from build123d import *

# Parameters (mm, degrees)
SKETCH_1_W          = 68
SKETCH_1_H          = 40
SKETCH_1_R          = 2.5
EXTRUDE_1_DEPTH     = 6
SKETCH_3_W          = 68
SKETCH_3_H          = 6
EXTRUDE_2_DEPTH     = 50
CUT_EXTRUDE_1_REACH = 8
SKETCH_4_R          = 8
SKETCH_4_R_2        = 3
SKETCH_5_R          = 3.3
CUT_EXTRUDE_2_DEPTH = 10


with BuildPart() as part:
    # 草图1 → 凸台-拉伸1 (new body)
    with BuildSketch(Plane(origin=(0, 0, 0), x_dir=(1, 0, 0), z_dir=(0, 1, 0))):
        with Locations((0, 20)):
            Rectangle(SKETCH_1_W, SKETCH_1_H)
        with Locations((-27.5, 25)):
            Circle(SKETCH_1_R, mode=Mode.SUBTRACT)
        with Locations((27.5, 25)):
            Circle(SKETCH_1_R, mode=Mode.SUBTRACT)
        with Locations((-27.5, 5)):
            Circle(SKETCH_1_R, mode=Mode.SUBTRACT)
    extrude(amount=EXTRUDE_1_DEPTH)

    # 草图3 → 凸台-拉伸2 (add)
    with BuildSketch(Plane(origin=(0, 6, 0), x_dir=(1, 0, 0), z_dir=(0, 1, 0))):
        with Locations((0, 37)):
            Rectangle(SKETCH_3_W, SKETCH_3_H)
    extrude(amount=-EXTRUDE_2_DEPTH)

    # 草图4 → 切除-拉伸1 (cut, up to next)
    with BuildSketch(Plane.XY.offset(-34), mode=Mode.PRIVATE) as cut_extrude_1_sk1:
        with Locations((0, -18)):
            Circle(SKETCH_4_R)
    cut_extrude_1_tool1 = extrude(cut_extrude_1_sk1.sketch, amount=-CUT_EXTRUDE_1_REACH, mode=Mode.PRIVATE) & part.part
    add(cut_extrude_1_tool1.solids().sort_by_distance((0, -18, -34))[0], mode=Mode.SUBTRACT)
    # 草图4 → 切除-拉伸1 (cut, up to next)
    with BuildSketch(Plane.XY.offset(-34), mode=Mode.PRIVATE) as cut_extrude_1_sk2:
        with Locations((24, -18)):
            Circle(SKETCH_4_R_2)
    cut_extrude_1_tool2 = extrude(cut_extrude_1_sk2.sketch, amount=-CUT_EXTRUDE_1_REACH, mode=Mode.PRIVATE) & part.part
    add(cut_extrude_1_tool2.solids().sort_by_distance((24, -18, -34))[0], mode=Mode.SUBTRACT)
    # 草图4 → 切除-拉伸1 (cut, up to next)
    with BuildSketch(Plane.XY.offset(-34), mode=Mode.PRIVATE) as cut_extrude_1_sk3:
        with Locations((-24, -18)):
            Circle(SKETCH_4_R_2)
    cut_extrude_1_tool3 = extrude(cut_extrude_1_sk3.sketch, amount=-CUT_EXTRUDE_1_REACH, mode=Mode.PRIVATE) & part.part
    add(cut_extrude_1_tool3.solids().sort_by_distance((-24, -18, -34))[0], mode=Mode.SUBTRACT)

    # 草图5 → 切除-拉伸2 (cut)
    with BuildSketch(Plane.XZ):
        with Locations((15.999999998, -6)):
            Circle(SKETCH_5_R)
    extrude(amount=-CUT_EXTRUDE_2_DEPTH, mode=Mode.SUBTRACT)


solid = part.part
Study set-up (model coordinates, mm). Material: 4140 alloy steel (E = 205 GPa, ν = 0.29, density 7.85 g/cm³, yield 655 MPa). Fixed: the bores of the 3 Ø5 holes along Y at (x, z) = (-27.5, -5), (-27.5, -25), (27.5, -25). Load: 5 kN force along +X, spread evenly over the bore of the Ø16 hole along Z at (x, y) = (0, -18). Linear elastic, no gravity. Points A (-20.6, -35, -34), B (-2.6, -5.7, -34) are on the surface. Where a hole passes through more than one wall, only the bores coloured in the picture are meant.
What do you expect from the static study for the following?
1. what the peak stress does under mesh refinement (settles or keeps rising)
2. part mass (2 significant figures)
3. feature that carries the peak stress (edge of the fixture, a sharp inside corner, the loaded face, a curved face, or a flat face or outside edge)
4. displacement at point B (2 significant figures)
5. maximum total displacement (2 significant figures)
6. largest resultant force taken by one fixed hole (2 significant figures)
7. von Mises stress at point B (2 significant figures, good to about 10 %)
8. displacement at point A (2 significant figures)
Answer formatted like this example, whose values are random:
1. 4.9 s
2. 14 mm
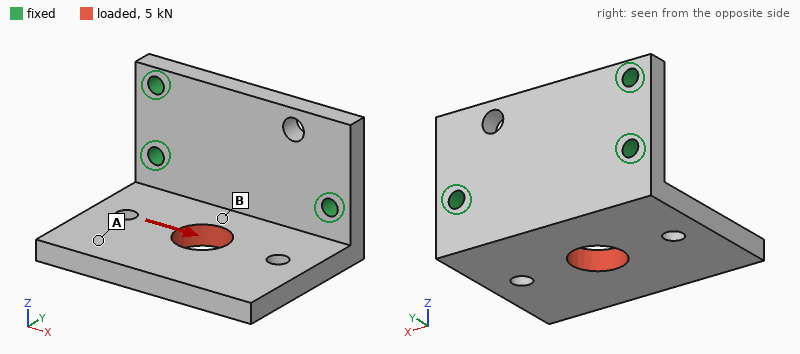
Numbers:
1. keeps rising
2. 250 g
3. edge of the fixture
4. 7.9 µm
5. 39 µm
6. 3.2 kN
7. 59 MPa
8. 29 µm
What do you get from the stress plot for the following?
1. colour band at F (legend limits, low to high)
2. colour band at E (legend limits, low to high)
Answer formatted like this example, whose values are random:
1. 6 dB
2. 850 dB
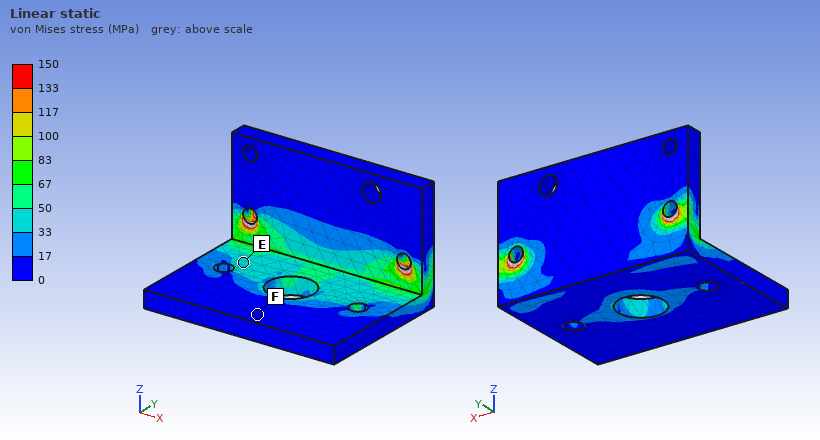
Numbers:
1. 0 to 17 MPa
2. 33 to 50 MPa
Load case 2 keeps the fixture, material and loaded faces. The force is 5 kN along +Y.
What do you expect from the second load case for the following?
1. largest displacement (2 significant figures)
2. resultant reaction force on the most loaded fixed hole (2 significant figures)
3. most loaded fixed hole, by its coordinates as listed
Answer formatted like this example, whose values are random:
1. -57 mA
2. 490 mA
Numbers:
1. 95 µm
2. 3.0 kN
3. (-27.5, -25)
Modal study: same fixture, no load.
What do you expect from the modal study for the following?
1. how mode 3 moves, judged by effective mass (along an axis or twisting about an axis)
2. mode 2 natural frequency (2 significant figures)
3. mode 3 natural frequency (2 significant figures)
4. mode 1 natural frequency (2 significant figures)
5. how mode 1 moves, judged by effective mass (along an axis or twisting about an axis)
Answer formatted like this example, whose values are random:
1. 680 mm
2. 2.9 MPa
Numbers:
1. along X
2. 3400 Hz
3. 6100 Hz
4. 1500 Hz
5. along Z
